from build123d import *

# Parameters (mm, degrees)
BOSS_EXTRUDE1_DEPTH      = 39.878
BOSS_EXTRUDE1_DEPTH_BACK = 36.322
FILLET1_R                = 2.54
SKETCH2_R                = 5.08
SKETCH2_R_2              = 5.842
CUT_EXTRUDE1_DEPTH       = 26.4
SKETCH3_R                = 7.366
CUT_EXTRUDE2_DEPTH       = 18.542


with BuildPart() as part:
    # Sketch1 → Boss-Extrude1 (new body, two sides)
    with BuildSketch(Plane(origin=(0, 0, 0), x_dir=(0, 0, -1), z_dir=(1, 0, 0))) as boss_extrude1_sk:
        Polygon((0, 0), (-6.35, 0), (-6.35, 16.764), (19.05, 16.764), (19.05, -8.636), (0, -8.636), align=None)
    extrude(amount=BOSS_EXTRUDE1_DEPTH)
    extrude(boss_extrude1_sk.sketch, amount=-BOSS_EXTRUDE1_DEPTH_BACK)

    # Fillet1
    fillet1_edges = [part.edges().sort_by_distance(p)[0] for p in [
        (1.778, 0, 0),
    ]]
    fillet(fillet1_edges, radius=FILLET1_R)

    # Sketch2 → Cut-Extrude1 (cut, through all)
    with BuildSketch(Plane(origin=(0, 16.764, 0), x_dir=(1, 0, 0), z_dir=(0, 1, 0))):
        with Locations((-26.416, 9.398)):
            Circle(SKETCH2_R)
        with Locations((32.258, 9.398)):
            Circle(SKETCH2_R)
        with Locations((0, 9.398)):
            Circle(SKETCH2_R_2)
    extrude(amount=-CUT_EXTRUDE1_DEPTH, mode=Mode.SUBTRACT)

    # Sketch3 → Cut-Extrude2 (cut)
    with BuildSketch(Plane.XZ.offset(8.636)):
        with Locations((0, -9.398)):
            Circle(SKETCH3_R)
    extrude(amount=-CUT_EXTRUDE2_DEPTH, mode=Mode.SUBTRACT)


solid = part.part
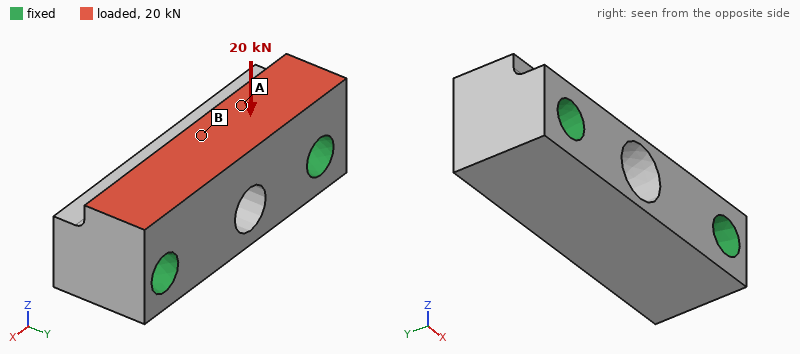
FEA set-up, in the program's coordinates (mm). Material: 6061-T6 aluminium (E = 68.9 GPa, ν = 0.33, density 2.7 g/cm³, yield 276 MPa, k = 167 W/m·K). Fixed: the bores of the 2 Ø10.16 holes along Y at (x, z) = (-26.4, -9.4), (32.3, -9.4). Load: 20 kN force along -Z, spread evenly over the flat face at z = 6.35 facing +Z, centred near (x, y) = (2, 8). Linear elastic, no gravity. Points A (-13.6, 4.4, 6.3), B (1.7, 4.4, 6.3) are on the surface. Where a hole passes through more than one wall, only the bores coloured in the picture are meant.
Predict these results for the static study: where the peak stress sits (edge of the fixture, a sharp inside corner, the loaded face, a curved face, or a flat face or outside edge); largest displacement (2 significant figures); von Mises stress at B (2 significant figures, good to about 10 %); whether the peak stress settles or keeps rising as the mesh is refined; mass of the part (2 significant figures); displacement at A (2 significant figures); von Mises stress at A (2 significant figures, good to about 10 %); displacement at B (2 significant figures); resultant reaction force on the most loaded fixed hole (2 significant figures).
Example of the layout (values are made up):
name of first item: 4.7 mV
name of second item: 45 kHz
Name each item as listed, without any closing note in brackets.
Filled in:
where the peak stress sits: edge of the fixture
largest displacement: 20 µm
von Mises stress at B: 32 MPa
whether the peak stress settles or keeps rising as the mesh is refined: keeps rising
mass of the part: 100 g
displacement at A: 9.5 µm
von Mises stress at A: 14 MPa
displacement at B: 15 µm
resultant reaction force on the most loaded fixed hole: 10 kN
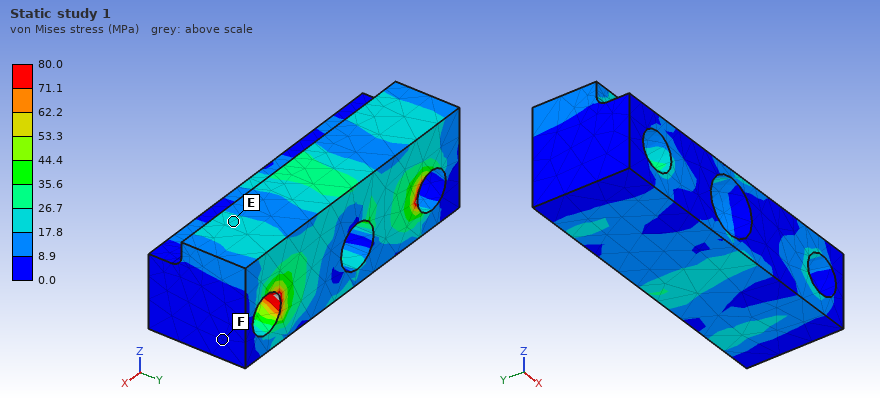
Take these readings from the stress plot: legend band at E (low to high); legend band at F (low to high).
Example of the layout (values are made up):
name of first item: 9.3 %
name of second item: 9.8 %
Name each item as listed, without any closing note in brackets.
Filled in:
legend band at E: 17.8 to 26.7 MPa
legend band at F: 0.0 to 8.9 MPa
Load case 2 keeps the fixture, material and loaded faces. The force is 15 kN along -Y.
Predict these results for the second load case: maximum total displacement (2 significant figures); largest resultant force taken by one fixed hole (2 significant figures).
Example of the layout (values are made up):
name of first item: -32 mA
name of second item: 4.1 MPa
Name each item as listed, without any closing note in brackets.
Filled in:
maximum total displacement: 33 µm
largest resultant force taken by one fixed hole: 7.7 kN
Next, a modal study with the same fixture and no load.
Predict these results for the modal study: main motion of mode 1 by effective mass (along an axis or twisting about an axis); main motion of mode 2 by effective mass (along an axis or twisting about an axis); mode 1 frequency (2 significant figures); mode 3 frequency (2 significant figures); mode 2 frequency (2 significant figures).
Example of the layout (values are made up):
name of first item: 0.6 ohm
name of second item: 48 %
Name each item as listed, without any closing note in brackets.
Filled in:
main motion of mode 1 by effective mass: along Z
main motion of mode 2 by effective mass: along Y
mode 1 frequency: 22 kHz
mode 3 frequency: 28 kHz
mode 2 frequency: 24 kHz
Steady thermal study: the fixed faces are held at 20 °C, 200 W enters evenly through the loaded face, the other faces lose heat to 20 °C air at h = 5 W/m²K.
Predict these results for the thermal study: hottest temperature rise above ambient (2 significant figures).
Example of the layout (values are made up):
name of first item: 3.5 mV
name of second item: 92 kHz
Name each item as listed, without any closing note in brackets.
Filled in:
hottest temperature rise above ambient: 22 K
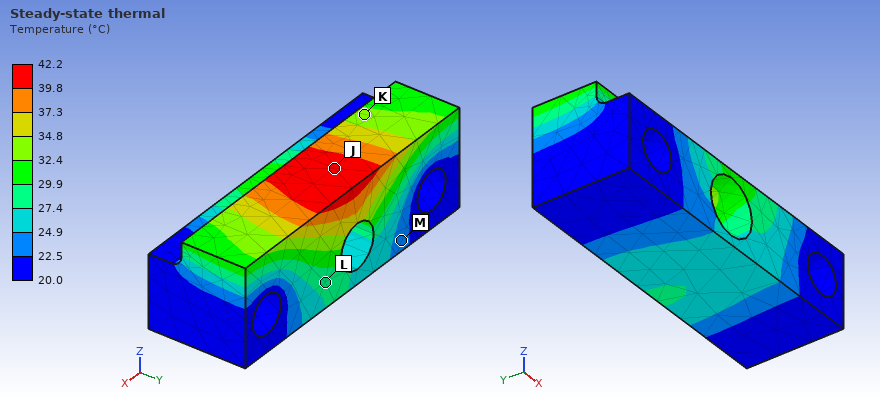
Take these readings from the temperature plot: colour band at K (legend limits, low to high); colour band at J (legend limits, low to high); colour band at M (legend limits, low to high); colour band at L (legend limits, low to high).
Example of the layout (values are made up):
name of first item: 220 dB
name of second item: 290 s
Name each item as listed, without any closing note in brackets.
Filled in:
colour band at K: 32.4 to 34.8 °C
colour band at J: 39.8 to 42.2 °C
colour band at M: 22.5 to 24.9 °C
colour band at L: 27.4 to 29.9 °C
